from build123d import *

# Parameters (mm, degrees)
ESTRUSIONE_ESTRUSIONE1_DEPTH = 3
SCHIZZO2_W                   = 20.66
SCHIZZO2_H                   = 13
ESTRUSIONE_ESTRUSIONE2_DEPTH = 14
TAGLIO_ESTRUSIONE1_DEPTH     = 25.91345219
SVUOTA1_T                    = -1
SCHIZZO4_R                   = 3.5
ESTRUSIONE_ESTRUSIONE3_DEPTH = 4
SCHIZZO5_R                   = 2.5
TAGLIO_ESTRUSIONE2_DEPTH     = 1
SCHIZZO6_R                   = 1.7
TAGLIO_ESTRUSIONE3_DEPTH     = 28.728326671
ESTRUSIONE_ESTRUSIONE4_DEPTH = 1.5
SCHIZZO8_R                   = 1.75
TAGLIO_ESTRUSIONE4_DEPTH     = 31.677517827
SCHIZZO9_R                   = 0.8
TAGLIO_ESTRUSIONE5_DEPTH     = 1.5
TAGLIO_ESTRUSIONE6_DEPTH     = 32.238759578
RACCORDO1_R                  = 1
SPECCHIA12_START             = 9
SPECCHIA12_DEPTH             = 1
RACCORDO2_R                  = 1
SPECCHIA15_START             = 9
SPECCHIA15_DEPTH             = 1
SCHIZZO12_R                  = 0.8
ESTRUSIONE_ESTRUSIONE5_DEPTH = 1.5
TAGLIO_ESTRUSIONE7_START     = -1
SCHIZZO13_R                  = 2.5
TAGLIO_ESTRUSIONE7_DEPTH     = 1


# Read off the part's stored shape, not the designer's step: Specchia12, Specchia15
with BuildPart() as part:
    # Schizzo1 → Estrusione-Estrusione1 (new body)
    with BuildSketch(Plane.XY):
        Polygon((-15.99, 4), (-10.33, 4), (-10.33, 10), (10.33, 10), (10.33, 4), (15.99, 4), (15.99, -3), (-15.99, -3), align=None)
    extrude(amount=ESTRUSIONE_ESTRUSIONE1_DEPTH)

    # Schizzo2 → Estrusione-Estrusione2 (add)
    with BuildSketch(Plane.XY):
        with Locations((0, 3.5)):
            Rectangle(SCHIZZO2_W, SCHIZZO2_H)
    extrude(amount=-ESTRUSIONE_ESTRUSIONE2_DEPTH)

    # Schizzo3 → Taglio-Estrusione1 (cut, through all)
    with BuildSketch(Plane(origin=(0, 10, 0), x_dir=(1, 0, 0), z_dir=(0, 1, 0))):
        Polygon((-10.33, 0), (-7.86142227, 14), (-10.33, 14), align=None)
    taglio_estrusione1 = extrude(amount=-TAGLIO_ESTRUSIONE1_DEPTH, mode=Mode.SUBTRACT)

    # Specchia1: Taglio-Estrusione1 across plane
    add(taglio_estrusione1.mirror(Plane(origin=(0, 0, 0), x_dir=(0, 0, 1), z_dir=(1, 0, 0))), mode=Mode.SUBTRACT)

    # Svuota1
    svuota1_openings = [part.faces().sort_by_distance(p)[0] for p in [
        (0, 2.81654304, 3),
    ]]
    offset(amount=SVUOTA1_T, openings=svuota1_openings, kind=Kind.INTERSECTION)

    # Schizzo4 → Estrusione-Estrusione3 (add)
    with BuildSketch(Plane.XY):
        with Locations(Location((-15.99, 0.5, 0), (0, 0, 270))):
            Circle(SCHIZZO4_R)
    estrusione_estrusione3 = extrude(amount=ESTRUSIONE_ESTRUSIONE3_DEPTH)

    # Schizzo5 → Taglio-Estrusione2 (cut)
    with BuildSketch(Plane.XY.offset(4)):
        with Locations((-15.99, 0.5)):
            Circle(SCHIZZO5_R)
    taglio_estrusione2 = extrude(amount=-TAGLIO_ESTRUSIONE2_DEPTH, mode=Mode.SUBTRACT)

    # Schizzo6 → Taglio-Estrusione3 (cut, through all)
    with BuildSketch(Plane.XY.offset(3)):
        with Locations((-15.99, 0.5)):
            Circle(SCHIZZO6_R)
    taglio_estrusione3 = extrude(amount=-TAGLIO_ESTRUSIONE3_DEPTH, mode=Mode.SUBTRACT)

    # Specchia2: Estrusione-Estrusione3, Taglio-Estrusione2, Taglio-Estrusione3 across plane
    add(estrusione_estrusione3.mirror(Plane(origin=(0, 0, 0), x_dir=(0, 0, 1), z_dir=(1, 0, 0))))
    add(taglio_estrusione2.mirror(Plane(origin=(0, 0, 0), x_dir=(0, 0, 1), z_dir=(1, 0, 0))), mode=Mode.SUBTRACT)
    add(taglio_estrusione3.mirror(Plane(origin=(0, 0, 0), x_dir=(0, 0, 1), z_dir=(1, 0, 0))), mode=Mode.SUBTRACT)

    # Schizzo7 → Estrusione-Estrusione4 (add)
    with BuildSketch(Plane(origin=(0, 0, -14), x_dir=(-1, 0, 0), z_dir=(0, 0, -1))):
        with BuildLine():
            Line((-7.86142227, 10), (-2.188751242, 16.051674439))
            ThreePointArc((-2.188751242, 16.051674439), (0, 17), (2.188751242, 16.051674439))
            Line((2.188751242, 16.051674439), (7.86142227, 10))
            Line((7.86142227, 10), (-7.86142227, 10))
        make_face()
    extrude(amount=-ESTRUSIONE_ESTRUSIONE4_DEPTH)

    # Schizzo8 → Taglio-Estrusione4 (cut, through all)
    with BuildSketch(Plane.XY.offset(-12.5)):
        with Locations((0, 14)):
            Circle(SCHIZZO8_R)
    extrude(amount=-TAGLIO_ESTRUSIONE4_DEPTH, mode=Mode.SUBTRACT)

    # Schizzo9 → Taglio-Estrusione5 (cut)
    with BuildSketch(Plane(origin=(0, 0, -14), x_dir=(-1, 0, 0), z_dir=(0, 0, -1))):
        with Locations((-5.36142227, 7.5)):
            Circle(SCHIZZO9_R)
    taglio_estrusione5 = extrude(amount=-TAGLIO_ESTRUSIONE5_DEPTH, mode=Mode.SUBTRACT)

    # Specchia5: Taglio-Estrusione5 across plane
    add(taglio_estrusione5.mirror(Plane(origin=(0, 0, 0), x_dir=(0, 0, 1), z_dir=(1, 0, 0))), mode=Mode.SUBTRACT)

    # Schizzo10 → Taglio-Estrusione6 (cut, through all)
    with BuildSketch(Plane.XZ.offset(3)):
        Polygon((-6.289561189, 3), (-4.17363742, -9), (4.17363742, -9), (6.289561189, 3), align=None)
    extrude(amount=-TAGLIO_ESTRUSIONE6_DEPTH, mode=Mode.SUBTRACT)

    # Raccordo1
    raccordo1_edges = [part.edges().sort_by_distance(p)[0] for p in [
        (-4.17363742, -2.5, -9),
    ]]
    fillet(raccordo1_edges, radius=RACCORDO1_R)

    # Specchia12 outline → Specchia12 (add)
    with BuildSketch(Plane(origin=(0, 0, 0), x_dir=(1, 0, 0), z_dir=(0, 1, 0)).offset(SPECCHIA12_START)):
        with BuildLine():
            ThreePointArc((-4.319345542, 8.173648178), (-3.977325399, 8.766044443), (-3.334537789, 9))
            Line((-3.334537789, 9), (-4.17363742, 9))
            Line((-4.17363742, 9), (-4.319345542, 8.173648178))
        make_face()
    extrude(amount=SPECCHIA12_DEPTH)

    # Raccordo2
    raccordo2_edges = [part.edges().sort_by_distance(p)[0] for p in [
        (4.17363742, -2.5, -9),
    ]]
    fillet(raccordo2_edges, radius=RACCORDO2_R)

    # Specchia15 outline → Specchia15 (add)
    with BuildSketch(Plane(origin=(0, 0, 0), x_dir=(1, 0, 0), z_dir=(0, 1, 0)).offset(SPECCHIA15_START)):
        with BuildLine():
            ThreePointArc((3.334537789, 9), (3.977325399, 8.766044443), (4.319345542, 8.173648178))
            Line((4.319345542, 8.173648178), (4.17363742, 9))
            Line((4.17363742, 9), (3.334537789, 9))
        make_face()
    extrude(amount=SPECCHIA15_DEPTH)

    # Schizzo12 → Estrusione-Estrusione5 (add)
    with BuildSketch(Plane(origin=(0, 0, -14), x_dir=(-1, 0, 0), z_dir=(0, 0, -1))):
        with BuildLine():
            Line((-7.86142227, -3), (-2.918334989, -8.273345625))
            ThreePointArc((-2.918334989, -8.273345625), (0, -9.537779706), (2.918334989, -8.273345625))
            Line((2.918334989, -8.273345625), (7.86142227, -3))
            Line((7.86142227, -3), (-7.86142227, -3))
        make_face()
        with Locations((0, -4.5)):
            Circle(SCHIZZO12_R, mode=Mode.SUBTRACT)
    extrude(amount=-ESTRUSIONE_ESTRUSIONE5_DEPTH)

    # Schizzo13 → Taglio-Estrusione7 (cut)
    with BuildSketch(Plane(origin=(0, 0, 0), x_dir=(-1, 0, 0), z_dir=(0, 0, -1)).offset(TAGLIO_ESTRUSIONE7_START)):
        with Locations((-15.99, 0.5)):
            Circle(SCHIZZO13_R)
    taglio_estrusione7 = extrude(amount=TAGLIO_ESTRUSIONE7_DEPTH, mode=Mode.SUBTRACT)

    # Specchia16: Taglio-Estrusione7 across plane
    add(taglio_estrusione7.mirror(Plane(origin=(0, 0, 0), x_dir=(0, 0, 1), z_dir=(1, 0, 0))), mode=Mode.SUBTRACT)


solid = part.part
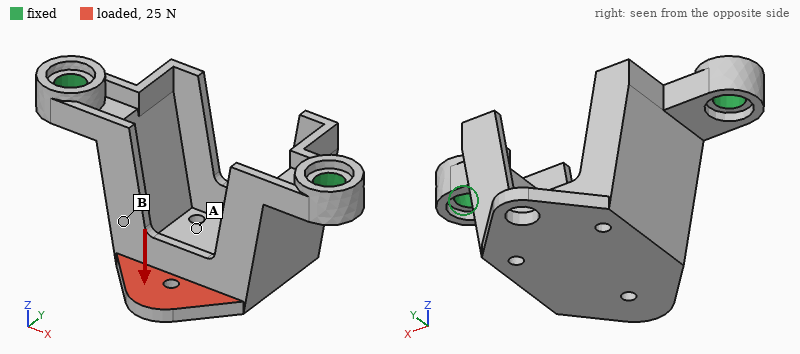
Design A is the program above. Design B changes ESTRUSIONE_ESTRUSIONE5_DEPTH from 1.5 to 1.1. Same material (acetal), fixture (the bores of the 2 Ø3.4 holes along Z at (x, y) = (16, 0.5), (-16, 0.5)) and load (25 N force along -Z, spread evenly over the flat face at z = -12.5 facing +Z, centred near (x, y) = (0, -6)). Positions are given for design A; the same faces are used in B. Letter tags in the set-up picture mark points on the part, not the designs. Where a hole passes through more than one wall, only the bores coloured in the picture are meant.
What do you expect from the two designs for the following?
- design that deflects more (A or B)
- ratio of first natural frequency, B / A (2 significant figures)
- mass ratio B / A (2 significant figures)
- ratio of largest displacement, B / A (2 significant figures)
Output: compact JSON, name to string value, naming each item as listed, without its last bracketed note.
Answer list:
{"design that deflects more": "B", "ratio of first natural frequency, B / A": "1.0", "mass ratio B / A": "0.98", "ratio of largest displacement, B / A": "1.3"}
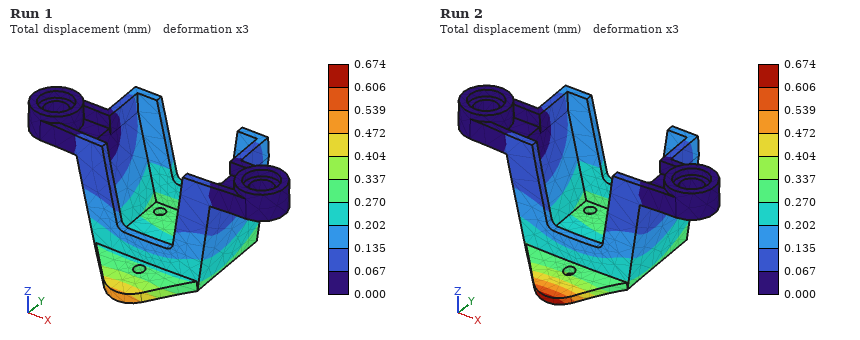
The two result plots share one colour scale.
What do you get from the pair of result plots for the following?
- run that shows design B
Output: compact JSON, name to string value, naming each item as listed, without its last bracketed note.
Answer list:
{"run that shows design B": "Run 2"}
